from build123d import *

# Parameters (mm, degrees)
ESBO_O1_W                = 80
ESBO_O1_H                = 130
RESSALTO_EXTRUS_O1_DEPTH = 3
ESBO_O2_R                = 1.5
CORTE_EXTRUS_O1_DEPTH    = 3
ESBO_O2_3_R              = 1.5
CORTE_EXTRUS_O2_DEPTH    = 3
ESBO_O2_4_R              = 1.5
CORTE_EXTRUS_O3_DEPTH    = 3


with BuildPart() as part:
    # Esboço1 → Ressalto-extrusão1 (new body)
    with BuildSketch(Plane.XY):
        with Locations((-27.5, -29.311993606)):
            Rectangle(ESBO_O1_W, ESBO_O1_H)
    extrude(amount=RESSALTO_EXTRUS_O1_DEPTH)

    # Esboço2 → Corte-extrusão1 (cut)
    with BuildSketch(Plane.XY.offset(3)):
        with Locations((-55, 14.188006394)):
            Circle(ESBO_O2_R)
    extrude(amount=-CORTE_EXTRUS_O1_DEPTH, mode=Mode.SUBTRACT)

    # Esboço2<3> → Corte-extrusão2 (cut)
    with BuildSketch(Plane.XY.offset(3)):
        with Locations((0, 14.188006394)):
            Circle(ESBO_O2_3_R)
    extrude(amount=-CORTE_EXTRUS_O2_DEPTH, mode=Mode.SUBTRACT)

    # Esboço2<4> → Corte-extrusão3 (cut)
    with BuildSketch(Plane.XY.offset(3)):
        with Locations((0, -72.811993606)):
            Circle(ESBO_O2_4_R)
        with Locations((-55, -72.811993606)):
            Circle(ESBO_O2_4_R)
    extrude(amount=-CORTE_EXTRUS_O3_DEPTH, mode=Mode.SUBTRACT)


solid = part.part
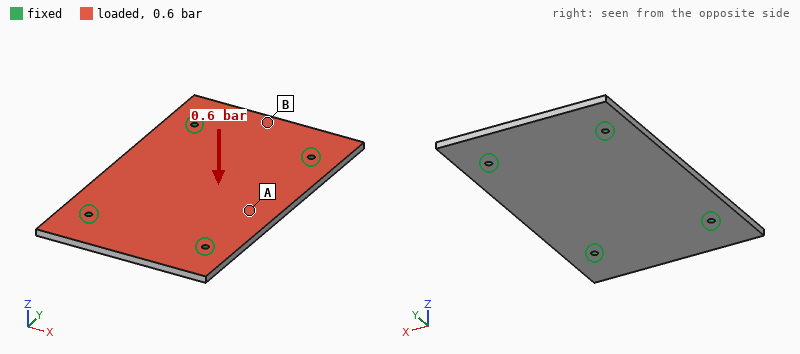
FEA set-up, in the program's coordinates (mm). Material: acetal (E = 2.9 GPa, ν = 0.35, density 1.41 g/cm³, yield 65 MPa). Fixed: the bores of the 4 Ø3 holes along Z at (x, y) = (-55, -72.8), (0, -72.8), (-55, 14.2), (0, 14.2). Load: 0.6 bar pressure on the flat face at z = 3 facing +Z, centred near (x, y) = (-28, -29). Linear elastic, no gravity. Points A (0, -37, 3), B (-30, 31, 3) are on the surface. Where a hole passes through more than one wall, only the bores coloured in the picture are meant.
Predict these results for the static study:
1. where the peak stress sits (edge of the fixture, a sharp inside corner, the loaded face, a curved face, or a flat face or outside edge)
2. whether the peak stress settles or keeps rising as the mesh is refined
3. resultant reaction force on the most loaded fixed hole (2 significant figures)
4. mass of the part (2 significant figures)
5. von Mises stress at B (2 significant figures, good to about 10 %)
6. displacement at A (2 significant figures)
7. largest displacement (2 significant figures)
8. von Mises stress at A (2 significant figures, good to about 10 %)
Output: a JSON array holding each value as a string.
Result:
["edge of the fixture", "keeps rising", "160 N", "44 g", "4.8 MPa", "1.6 mm", "1.8 mm", "12 MPa"]
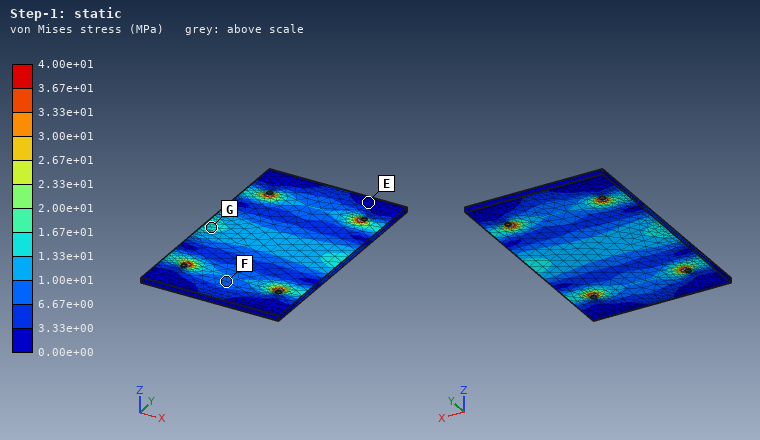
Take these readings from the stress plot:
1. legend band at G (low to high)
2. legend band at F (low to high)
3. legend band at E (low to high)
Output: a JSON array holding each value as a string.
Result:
["1.33e+01 to 1.67e+01 MPa", "6.67e+00 to 1.00e+01 MPa", "0.00e+00 to 3.33e+00 MPa"]
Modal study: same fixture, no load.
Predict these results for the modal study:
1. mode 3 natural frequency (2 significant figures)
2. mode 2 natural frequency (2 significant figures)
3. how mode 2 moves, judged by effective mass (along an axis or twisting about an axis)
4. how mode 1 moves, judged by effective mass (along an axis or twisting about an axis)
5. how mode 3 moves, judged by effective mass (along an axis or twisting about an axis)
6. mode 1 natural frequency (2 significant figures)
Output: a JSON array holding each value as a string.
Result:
["950 Hz", "680 Hz", "twisting about Y", "along Z", "along Z", "490 Hz"]
